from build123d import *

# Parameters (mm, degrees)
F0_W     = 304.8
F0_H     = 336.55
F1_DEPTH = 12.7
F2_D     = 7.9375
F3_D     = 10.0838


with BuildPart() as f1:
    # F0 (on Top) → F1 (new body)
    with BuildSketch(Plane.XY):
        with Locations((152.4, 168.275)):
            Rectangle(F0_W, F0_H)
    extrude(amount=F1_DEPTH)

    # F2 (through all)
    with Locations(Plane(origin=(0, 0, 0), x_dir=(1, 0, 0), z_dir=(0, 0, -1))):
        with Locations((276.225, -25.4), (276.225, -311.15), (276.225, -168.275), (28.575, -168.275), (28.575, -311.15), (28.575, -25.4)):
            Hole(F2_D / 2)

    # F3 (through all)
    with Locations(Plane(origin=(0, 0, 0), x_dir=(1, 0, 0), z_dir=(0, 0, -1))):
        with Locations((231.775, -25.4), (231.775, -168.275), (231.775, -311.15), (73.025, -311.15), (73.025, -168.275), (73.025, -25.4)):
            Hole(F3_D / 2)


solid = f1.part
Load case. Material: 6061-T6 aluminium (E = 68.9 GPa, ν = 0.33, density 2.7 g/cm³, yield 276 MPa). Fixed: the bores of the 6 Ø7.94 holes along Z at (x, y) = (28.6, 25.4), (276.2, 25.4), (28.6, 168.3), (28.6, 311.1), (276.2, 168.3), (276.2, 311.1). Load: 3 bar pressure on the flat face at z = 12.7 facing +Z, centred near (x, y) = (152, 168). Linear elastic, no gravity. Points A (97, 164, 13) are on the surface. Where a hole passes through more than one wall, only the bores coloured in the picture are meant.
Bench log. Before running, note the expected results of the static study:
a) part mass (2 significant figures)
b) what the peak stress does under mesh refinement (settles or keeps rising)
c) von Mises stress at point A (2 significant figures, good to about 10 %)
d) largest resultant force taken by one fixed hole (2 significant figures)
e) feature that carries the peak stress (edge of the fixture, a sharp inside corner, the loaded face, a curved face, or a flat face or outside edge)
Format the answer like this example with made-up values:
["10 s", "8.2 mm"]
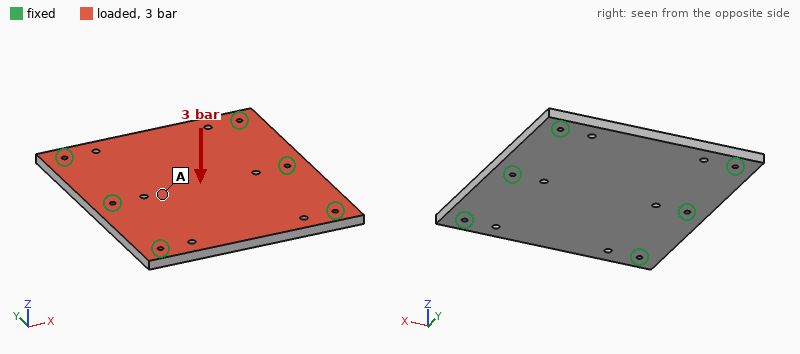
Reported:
["3.5 kg", "keeps rising", "21 MPa", "6.7 kN", "edge of the fixture"]
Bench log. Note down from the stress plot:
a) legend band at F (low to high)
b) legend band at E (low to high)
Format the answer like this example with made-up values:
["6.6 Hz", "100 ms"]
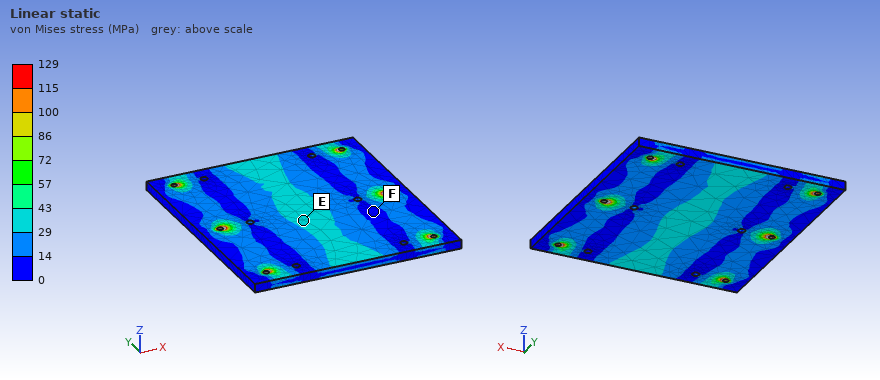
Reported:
["0 to 14 MPa", "29 to 43 MPa"]
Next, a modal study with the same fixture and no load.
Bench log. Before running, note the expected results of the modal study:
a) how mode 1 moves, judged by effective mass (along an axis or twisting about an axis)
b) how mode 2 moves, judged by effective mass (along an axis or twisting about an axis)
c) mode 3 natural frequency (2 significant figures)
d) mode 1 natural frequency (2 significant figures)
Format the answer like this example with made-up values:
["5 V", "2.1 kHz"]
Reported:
["along Z", "twisting about X", "1500 Hz", "860 Hz"]
